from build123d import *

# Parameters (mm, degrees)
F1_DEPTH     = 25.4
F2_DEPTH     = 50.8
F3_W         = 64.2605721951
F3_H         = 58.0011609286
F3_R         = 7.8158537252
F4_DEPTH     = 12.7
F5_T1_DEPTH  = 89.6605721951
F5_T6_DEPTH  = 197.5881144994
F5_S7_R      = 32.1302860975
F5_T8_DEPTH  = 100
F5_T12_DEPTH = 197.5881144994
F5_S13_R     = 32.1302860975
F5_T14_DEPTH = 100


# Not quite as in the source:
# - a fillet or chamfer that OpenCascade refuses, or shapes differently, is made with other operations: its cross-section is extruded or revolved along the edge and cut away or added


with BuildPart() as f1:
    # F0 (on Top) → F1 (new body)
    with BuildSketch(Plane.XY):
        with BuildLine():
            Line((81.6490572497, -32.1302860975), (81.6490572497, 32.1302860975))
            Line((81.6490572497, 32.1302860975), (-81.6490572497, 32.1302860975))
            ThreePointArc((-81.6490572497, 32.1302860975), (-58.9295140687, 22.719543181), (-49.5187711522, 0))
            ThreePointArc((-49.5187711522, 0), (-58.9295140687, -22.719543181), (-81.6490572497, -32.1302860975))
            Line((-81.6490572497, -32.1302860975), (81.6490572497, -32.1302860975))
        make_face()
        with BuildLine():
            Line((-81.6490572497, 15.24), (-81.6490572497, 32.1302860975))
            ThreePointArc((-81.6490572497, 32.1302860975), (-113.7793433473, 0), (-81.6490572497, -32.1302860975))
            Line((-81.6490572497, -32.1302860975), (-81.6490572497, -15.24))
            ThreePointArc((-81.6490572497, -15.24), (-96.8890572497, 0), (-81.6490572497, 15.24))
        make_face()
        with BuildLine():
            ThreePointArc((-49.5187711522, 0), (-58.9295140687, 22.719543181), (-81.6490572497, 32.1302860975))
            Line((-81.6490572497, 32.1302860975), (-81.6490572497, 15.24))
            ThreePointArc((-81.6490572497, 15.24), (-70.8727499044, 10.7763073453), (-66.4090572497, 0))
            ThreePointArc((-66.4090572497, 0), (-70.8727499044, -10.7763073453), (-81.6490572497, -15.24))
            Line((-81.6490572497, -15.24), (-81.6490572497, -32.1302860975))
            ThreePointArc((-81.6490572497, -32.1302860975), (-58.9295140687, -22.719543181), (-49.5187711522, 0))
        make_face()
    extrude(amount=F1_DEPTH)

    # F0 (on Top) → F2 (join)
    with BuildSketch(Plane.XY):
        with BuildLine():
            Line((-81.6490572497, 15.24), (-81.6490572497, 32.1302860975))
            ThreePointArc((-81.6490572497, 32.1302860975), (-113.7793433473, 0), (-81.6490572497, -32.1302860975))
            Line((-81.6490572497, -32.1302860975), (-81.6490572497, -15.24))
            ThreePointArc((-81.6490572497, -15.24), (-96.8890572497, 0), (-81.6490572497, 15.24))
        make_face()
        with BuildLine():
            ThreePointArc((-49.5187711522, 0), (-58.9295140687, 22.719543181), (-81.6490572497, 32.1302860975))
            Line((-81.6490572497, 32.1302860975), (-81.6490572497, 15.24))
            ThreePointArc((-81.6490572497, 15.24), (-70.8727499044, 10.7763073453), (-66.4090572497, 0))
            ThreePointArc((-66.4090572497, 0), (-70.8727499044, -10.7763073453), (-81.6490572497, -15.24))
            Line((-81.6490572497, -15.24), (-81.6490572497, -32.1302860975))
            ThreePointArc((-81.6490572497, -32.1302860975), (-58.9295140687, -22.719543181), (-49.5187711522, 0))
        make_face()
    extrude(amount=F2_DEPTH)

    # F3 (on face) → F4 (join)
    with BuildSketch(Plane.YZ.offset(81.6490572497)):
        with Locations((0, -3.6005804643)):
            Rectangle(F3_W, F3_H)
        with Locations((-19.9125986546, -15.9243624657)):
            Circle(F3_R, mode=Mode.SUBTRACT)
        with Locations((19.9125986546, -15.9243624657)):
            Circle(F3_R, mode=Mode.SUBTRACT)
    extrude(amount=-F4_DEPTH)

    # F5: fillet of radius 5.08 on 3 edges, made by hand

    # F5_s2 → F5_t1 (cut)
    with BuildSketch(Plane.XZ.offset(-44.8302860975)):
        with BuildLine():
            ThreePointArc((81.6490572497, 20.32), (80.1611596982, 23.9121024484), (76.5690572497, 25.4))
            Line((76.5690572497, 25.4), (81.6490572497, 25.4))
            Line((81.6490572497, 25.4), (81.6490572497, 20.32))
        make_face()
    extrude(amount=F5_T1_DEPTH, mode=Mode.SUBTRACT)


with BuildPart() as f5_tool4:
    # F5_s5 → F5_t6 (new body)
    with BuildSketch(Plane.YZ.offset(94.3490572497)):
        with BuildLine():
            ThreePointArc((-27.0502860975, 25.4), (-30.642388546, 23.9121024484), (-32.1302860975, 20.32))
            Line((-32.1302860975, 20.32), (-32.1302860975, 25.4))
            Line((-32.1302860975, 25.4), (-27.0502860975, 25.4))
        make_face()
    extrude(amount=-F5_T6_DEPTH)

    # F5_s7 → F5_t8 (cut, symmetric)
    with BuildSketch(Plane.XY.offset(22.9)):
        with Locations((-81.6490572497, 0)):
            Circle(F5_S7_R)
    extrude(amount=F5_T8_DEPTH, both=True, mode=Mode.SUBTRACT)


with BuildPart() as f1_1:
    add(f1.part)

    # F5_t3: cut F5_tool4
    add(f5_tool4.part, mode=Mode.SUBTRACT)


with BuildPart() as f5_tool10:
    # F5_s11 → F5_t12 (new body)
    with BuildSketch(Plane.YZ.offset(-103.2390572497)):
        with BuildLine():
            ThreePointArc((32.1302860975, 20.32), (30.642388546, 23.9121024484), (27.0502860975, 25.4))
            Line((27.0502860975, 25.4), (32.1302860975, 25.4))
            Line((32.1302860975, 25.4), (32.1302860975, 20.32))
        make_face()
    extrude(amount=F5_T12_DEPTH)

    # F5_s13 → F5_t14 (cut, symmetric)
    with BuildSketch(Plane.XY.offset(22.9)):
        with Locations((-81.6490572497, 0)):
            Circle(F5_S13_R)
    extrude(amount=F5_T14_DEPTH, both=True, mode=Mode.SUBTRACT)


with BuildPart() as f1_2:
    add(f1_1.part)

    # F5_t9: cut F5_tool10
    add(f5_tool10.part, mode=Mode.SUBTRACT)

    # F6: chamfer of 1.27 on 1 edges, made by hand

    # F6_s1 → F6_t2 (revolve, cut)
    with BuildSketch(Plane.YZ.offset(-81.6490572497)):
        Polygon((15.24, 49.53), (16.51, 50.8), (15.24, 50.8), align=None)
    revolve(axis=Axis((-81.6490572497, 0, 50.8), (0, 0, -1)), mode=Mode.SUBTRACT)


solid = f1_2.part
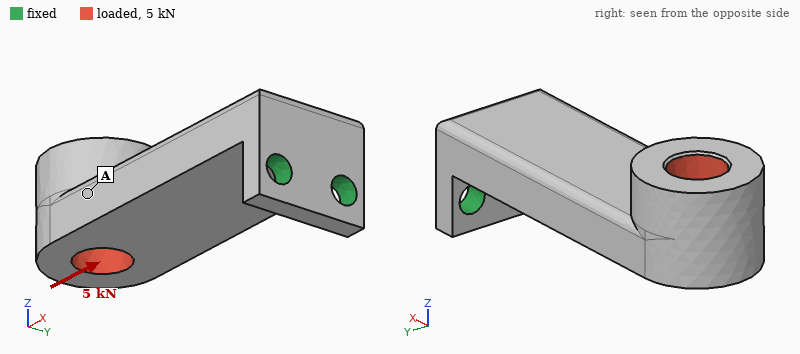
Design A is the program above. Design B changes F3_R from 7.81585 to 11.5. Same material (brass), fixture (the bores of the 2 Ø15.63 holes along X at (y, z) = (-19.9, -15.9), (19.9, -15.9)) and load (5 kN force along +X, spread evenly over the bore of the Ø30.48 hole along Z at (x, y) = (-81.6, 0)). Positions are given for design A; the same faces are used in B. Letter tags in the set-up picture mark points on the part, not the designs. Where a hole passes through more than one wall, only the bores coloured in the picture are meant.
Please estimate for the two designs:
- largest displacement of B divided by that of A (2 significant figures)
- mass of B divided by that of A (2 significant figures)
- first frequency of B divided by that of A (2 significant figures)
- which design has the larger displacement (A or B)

0.76
0.98
1.1
A
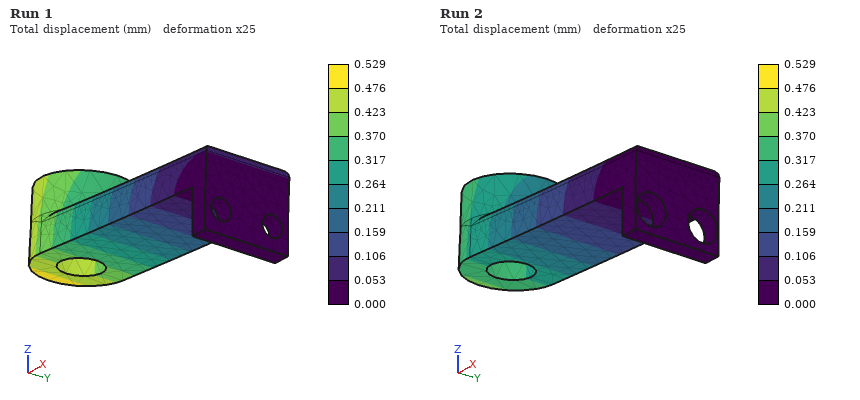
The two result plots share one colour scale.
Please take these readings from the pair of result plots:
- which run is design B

Run 2
